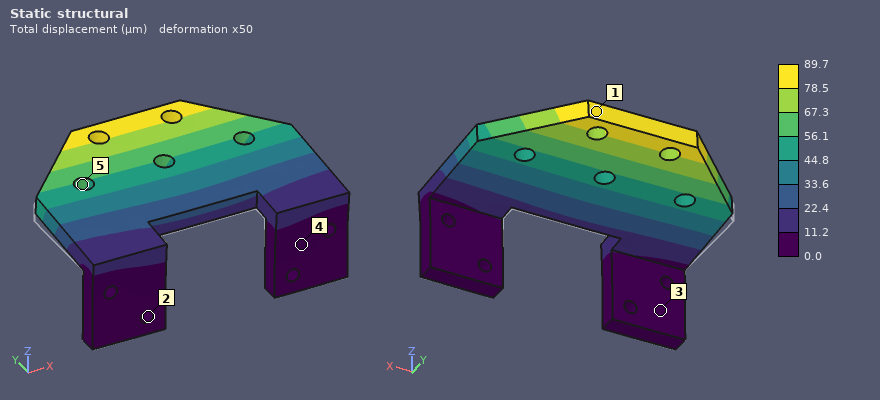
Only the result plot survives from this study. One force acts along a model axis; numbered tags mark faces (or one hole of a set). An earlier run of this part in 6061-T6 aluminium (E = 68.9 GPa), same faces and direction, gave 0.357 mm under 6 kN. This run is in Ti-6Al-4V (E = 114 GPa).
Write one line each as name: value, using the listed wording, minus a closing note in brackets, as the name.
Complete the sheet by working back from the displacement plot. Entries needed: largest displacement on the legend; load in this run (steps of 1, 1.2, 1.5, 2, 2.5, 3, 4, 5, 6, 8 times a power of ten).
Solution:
largest displacement on the legend: 89.7 µm
load in this run: 2.5 kN
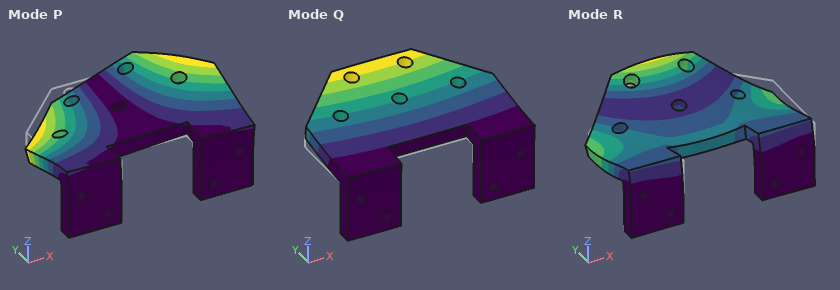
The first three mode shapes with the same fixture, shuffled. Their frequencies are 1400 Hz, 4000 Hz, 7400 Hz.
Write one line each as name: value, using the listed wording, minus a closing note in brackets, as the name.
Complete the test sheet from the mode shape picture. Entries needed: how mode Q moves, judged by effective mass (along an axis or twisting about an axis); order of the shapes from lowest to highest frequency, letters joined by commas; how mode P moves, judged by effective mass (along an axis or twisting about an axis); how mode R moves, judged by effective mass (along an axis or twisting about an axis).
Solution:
how mode Q moves, judged by effective mass: along Z
order of the shapes from lowest to highest frequency, letters joined by commas: Q, P, R
how mode P moves, judged by effective mass: twisting about Y
how mode R moves, judged by effective mass: along Y
